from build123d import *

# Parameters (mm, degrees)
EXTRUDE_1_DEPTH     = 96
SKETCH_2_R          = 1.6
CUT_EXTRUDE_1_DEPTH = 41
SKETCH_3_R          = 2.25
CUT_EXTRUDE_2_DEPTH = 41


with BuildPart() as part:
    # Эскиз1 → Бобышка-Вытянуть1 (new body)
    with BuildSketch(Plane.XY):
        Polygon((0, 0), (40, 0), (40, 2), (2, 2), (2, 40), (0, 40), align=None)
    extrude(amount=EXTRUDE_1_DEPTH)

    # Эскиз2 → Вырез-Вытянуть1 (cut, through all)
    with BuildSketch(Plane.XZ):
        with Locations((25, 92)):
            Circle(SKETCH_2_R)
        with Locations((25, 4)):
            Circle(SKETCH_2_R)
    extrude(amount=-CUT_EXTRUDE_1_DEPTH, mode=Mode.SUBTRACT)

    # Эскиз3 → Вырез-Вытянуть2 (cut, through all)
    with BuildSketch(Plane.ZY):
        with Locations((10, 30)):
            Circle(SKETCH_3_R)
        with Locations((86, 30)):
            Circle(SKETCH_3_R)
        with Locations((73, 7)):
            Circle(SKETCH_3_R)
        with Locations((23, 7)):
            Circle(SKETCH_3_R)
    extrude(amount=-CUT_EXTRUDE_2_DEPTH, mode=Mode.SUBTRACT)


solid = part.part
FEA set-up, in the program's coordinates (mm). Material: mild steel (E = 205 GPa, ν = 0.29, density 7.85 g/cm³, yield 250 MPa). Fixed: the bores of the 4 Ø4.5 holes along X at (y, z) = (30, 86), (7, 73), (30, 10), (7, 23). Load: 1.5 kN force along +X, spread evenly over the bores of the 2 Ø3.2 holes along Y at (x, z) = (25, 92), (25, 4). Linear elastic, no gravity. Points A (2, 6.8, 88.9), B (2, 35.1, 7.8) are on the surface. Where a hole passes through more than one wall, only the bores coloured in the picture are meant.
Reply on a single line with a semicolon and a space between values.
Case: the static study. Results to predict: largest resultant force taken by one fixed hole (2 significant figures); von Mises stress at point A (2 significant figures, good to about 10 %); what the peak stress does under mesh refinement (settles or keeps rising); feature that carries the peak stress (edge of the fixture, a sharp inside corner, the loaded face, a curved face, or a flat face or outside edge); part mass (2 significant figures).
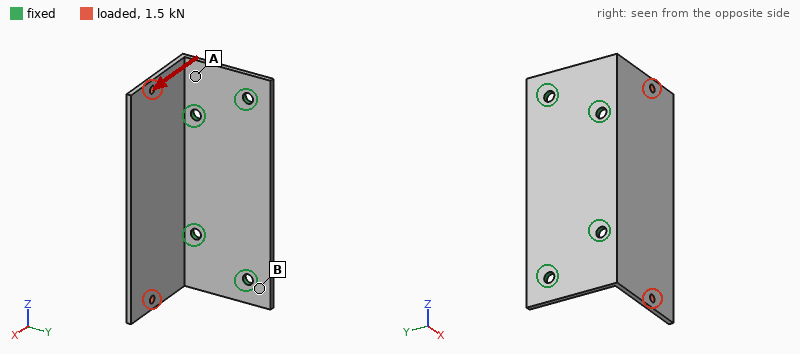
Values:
860 N; 31 MPa; keeps rising; edge of the fixture; 120 g
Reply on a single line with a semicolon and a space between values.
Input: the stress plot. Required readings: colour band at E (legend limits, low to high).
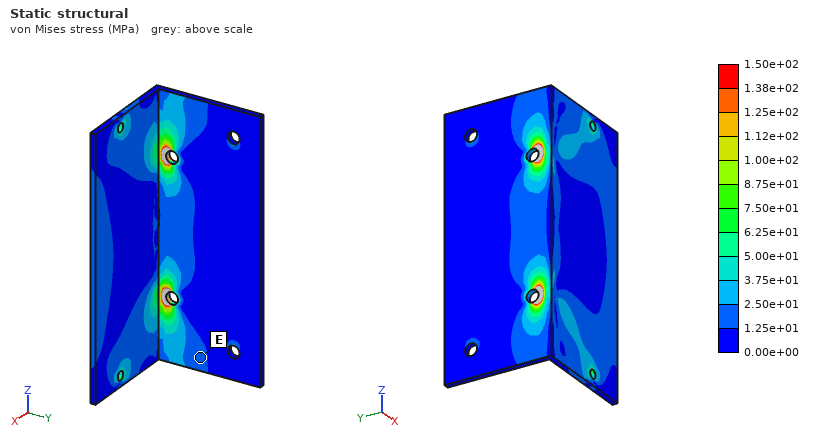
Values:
1.25e+01 to 2.50e+01 MPa
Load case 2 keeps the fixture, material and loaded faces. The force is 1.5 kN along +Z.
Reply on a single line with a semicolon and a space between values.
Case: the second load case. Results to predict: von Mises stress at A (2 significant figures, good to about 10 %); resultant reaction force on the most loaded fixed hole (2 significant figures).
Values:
19 MPa; 980 N
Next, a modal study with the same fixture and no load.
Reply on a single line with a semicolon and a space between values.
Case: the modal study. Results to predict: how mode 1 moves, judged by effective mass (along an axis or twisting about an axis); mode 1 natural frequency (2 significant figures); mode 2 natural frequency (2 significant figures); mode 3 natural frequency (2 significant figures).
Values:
along Y; 860 Hz; 1300 Hz; 2400 Hz
